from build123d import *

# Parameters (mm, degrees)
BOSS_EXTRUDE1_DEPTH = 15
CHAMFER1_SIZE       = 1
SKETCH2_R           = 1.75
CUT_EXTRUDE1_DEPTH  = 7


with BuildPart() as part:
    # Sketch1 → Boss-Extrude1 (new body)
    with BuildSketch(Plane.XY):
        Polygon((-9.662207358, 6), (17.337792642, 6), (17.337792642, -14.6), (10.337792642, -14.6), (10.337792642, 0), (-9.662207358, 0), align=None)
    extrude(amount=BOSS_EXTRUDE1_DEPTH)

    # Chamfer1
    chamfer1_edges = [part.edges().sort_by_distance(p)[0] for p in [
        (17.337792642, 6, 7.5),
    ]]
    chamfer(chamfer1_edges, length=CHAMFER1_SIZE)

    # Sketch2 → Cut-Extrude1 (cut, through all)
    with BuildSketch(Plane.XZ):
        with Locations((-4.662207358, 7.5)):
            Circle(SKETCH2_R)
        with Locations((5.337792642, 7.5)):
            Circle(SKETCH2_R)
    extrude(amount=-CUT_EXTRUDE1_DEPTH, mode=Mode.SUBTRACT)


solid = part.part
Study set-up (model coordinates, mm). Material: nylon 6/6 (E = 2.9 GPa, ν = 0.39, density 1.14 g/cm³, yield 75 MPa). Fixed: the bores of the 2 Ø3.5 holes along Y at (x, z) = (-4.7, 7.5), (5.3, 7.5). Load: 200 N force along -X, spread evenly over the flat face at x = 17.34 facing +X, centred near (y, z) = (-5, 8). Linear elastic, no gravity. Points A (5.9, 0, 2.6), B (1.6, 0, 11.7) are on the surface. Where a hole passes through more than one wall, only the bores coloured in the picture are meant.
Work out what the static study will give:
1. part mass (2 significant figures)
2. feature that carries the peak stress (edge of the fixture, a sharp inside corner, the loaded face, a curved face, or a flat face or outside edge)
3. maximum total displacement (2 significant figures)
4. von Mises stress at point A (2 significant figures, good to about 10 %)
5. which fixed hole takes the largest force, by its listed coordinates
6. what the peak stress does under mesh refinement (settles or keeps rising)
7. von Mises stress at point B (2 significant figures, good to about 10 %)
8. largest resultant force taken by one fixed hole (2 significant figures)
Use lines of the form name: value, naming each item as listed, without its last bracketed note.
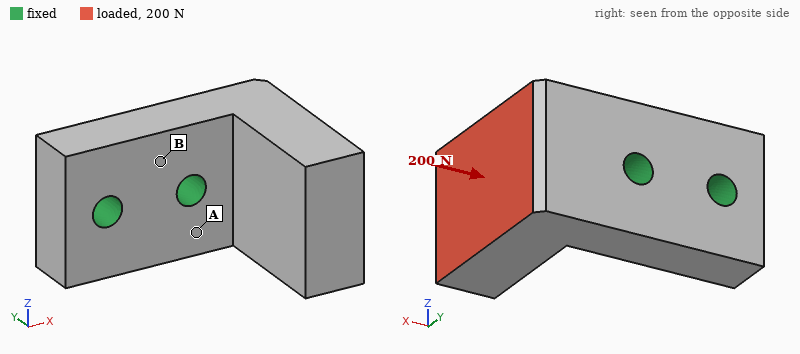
part mass: 4.4 g
feature that carries the peak stress: edge of the fixture
maximum total displacement: 0.36 mm
von Mises stress at point A: 11 MPa
which fixed hole takes the largest force, by its listed coordinates: (5.3, 7.5)
what the peak stress does under mesh refinement: keeps rising
von Mises stress at point B: 3.8 MPa
largest resultant force taken by one fixed hole: 170 N
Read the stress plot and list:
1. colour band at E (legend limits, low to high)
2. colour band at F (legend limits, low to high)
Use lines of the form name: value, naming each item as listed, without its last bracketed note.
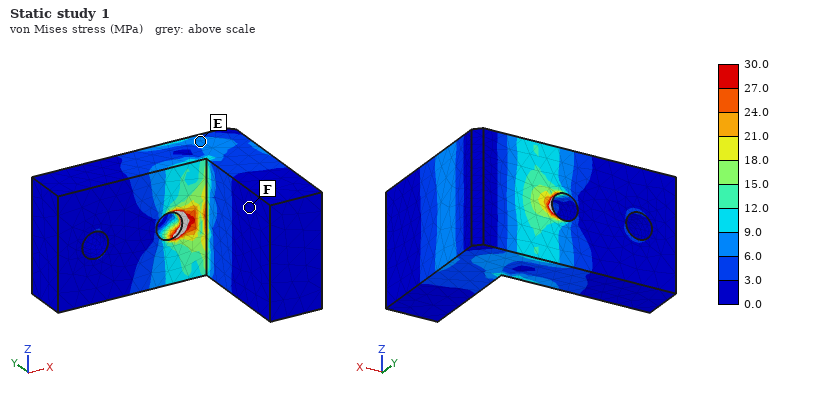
colour band at E: 6.0 to 9.0 MPa
colour band at F: 0.0 to 3.0 MPa
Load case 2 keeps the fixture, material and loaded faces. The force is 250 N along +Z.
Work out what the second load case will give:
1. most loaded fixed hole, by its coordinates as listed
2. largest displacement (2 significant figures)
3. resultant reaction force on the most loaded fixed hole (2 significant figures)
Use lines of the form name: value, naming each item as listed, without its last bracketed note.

most loaded fixed hole, by its coordinates as listed: (5.3, 7.5)
largest displacement: 0.36 mm
resultant reaction force on the most loaded fixed hole: 420 N
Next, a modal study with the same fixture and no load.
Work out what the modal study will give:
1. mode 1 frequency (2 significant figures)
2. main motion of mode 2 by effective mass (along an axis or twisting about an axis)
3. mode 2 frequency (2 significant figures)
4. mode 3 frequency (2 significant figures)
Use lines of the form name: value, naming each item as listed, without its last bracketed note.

mode 1 frequency: 2800 Hz
main motion of mode 2 by effective mass: along Z
mode 2 frequency: 3400 Hz
mode 3 frequency: 7400 Hz
